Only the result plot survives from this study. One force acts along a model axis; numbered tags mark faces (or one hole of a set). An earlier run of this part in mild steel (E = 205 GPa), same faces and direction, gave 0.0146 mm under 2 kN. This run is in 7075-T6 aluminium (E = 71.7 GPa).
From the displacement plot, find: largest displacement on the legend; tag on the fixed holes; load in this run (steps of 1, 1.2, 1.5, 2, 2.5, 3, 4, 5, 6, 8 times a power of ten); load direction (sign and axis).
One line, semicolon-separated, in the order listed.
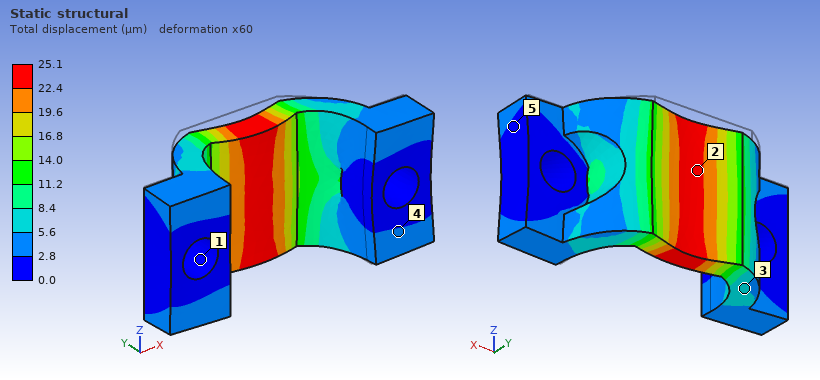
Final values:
25.1 µm; 1; 1.2 kN; -Y
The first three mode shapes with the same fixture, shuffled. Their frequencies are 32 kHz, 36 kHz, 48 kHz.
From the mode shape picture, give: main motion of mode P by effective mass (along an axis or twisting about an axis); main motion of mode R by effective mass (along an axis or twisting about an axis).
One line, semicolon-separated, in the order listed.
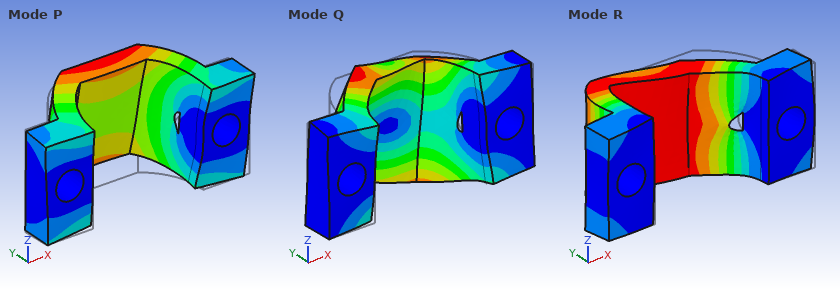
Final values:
along Z; along X
